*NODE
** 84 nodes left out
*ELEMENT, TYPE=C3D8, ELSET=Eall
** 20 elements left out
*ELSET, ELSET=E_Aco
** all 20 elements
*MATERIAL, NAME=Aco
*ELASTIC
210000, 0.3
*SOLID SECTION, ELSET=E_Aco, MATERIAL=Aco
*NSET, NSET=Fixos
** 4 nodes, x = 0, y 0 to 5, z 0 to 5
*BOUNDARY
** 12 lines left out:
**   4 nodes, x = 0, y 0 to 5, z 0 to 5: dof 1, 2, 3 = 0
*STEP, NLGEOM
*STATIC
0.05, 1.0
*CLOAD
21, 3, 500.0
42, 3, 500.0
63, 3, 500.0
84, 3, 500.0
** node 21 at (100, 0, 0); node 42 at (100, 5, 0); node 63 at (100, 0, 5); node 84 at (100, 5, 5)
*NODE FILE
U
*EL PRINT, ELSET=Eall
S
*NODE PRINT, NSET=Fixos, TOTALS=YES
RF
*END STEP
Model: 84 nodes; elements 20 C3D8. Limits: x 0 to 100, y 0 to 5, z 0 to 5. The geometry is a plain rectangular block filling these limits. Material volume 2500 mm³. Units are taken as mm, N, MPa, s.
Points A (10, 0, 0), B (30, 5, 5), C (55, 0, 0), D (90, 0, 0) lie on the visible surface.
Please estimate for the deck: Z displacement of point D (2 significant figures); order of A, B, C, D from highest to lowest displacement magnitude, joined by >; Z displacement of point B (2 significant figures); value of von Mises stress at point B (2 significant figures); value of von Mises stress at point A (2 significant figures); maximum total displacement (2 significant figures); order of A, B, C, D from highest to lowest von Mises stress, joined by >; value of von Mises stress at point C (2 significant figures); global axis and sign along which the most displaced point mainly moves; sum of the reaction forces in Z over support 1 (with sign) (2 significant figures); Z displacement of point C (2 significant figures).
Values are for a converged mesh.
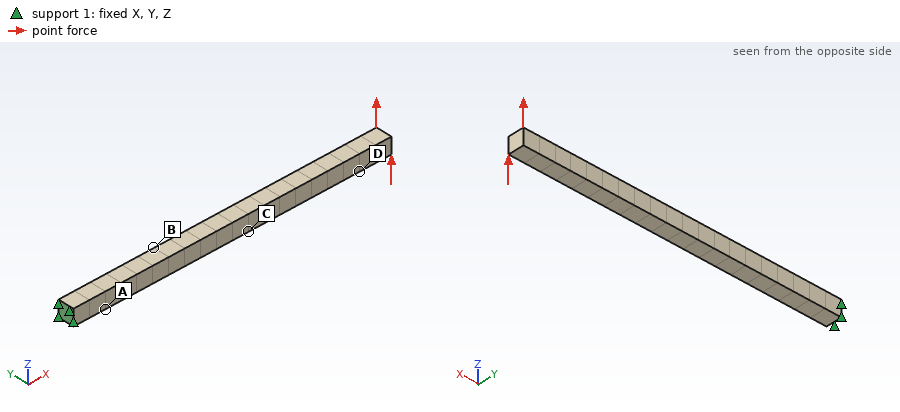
41 mm
D > C > B > A
5.9 mm
5200 MPa
7800 MPa
49 mm
A > B > C > D
3500 MPa
+Z
-2000 N
19 mm
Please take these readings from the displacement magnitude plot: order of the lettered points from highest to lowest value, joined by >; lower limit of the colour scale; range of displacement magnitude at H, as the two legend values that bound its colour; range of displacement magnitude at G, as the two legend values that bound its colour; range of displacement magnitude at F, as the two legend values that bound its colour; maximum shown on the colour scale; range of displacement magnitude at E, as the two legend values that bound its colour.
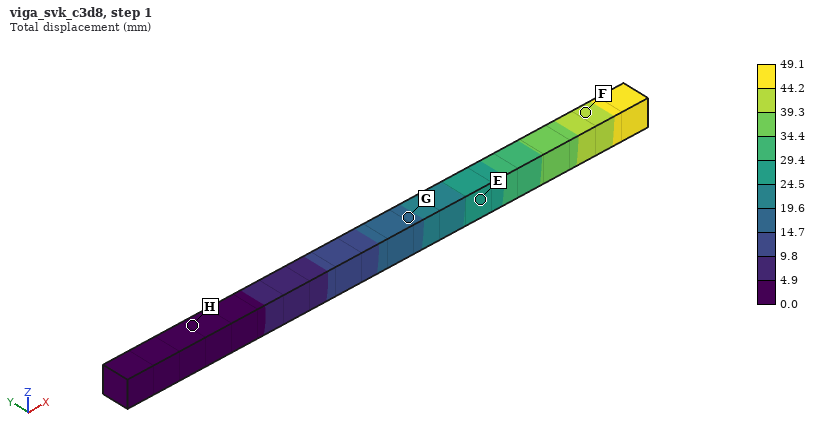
F > E > G > H
0.0 mm
0.0 to 4.9 mm
14.7 to 19.6 mm
39.3 to 44.2 mm
49.1 mm
24.5 to 29.4 mm
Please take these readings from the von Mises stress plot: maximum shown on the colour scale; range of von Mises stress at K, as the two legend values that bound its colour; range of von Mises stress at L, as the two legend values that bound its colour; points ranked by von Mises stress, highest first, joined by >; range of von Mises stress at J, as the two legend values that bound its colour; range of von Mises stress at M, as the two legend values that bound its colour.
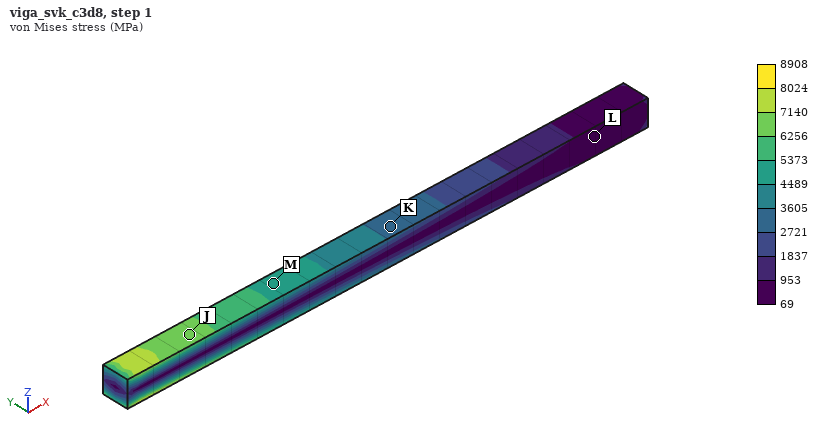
8908 MPa
2721 to 3605 MPa
69 to 953 MPa
J > M > K > L
6256 to 7140 MPa
4489 to 5373 MPa
